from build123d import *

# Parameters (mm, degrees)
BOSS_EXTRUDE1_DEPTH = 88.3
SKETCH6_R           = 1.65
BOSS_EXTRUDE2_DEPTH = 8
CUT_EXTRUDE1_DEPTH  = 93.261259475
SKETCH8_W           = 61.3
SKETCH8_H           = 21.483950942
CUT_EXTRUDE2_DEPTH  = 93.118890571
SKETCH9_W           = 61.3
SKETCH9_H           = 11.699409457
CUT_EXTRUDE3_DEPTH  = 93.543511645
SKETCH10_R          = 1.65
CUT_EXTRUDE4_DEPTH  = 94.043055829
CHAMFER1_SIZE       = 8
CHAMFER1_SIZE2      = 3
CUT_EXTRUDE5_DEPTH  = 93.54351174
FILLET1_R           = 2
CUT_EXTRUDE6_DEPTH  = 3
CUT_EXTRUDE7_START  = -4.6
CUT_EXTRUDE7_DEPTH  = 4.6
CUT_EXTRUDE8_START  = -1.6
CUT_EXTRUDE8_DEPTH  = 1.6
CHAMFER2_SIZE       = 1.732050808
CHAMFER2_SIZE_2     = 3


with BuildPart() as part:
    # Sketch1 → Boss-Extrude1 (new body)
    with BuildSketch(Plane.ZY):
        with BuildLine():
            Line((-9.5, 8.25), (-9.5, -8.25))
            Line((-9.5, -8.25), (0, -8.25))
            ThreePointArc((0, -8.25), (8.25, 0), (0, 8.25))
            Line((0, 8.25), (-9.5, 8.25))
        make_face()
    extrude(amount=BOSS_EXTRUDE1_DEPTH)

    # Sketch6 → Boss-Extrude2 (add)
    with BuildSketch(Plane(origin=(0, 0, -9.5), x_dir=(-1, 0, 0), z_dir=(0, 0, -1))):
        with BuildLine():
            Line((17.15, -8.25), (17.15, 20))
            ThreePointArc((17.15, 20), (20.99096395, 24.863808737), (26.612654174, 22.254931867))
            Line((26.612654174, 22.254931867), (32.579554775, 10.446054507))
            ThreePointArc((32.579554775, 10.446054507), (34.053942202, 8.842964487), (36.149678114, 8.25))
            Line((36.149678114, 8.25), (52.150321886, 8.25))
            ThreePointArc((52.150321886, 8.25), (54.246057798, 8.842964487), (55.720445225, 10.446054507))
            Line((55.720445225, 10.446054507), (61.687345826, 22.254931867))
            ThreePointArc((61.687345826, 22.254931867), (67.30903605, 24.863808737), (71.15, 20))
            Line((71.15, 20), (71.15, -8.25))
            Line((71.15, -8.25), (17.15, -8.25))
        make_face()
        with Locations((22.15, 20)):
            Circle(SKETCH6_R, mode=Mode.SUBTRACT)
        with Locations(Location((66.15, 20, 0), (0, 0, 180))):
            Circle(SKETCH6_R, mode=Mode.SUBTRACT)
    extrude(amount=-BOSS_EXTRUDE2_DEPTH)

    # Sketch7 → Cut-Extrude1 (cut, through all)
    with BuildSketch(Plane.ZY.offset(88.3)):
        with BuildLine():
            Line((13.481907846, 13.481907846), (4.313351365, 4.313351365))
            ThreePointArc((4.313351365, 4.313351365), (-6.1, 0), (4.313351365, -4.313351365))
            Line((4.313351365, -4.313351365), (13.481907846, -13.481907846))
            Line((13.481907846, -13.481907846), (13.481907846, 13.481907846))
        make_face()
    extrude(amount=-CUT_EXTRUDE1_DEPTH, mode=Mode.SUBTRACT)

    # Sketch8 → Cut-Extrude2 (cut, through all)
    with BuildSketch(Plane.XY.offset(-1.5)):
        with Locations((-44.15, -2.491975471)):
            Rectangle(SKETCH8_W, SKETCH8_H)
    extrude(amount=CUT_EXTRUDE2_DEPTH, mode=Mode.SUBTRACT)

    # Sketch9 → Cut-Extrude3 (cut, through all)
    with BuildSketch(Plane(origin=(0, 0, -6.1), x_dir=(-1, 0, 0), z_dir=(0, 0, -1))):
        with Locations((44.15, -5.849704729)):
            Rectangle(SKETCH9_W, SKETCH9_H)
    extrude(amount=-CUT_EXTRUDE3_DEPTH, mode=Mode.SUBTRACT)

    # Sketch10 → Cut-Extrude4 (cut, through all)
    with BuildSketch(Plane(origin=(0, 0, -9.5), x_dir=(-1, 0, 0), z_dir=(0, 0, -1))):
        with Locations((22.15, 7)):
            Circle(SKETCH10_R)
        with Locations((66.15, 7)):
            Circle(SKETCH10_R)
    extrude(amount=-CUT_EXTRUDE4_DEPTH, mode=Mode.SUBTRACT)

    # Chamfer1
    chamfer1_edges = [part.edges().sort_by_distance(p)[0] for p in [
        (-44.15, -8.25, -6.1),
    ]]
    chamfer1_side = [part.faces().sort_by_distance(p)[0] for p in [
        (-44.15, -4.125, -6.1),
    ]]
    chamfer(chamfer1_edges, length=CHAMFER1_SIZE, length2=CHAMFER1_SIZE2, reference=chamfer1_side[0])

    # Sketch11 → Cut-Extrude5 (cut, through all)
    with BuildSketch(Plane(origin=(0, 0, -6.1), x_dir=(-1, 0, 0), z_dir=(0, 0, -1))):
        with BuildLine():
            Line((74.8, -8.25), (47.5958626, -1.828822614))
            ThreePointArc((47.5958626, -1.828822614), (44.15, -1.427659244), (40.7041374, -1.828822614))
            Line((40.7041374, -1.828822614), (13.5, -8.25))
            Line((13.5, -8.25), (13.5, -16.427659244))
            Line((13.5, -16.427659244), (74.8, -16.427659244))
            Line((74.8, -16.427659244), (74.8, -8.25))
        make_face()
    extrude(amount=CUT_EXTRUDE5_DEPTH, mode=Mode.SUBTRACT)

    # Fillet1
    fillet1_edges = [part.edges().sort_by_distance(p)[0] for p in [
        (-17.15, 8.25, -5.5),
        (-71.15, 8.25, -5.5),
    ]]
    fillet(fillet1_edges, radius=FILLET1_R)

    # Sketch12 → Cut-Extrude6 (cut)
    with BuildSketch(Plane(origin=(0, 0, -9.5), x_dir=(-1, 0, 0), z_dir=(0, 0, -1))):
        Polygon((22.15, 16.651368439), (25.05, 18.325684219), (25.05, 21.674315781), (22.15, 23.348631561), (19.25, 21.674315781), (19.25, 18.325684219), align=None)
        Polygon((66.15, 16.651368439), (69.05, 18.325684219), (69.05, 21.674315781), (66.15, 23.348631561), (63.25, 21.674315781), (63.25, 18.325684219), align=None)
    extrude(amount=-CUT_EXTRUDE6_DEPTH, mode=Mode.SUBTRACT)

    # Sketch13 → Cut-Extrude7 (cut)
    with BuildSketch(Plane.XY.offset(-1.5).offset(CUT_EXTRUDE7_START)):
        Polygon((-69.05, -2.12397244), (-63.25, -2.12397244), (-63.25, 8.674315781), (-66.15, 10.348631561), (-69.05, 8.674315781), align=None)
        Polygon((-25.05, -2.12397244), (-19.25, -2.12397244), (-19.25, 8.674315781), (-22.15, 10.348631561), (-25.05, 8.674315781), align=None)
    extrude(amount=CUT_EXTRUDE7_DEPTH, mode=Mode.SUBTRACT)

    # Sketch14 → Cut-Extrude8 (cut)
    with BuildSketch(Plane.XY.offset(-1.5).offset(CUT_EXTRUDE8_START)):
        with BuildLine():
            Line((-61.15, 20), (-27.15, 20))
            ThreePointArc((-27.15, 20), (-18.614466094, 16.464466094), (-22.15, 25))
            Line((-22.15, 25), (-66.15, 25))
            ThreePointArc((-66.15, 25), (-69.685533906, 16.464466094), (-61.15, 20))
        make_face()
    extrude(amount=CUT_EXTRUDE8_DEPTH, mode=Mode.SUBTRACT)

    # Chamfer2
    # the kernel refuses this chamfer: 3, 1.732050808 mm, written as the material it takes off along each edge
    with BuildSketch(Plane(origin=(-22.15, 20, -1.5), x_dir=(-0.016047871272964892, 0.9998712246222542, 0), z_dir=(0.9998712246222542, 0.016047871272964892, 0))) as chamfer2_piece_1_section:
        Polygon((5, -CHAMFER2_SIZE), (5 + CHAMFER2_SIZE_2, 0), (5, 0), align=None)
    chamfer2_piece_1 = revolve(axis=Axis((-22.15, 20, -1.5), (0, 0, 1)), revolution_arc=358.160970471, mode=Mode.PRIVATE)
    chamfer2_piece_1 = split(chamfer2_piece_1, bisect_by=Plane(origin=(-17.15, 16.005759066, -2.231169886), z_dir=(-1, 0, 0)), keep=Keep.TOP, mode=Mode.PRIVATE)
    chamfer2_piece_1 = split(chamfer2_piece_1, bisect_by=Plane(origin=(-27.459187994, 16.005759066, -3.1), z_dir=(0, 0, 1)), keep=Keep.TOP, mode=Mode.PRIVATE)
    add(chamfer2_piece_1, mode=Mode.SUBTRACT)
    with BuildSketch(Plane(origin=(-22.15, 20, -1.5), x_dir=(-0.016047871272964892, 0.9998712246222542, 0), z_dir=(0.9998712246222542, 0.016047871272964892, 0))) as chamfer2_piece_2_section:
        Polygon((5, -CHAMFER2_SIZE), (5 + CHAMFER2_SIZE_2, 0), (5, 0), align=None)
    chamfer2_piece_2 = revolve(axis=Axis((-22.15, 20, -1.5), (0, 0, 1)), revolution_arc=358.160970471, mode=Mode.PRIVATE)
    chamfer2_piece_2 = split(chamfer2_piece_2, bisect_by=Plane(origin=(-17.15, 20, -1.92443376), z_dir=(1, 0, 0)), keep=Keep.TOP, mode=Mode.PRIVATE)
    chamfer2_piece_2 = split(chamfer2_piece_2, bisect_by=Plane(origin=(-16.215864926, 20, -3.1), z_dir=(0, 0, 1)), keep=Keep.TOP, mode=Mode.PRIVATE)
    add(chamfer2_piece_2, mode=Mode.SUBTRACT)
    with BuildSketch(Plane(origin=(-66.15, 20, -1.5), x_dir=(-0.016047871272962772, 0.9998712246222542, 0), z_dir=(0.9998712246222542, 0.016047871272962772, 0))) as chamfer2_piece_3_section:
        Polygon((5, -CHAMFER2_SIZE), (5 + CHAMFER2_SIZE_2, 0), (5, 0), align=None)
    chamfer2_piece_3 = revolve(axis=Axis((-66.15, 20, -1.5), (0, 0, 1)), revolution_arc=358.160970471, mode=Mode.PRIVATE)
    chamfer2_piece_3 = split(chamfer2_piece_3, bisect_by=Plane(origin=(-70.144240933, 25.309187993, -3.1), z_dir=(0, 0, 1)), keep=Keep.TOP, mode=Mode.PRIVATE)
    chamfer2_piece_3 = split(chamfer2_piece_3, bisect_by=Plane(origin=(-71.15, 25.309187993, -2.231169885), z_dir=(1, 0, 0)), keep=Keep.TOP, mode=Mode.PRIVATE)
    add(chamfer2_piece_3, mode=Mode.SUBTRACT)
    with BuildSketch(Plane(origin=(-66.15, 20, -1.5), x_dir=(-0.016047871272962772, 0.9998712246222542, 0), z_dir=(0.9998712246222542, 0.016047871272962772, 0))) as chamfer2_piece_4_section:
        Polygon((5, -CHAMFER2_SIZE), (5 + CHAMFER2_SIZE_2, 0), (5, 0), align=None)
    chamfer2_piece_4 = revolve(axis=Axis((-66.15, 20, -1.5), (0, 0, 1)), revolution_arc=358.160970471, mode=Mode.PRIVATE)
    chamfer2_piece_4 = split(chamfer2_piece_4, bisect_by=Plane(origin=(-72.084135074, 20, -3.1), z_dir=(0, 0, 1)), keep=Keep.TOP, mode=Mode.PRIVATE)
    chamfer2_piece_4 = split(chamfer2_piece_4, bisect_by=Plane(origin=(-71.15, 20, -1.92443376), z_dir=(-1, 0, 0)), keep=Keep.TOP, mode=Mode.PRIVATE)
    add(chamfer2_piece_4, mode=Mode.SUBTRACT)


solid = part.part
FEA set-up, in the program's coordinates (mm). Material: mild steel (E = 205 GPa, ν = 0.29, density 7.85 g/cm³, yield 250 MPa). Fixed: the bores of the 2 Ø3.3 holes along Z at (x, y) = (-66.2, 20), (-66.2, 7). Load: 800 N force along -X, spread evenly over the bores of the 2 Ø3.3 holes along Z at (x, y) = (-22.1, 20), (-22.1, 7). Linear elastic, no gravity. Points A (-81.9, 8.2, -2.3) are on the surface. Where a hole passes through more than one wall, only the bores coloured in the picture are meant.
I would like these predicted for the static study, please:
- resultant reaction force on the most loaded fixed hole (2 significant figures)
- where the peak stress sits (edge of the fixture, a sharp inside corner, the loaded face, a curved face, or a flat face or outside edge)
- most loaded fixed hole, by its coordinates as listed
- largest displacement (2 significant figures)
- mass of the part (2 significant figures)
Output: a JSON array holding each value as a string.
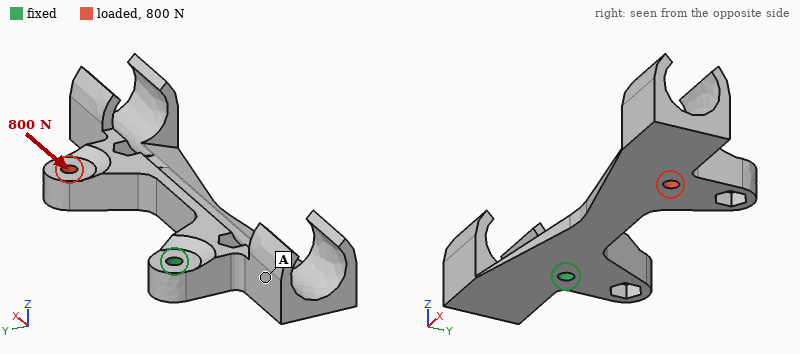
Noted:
["470 N", "a curved face", "(-66.2, 7)", "0.15 mm", "72 g"]
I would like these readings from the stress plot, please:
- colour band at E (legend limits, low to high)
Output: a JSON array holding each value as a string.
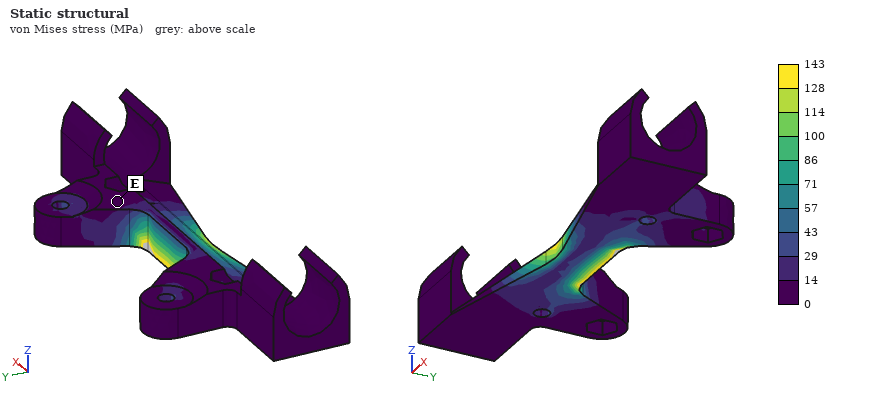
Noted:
["0 to 14 MPa"]
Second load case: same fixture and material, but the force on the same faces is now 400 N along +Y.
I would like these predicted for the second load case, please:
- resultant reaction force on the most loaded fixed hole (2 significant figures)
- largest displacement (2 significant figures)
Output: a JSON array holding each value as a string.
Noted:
["1.2 kN", "0.24 mm"]
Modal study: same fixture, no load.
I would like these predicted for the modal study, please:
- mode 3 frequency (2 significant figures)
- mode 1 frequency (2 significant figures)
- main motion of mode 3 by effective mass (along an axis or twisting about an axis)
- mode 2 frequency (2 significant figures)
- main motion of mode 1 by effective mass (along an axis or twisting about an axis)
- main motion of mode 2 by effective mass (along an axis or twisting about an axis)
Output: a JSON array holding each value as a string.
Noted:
["2600 Hz", "780 Hz", "twisting about X", "1500 Hz", "along Z", "along Y"]
